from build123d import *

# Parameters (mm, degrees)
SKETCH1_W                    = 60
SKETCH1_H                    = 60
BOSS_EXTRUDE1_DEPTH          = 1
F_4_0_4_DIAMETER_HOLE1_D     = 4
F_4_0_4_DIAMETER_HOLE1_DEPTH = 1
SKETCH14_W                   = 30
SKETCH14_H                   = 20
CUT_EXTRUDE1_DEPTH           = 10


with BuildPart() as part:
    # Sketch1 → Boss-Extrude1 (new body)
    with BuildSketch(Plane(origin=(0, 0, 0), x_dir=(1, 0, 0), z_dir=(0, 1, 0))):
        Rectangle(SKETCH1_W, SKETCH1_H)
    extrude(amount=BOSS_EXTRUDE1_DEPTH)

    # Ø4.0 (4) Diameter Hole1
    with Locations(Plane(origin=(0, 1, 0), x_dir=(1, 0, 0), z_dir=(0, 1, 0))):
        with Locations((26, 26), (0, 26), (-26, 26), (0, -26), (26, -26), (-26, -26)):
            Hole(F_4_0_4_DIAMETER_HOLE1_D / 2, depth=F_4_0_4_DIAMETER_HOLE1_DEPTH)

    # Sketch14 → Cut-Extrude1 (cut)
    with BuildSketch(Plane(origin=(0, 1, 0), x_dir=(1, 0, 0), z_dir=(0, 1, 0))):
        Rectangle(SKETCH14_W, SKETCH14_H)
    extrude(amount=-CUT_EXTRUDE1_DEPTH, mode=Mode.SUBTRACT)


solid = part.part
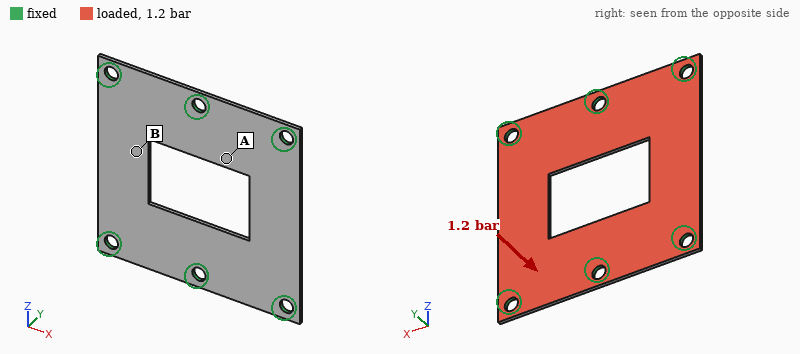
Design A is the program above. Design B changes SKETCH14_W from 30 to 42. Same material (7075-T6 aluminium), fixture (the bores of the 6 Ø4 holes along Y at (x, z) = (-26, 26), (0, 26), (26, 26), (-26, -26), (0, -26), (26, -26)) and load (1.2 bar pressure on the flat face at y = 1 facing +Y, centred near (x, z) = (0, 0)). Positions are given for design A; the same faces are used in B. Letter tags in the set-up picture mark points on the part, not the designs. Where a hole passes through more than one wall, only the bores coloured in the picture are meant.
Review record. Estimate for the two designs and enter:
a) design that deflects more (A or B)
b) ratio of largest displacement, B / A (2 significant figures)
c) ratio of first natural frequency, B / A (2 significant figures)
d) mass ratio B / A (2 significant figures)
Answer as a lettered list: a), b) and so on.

a) A
b) 0.88
c) 1.1
d) 0.92
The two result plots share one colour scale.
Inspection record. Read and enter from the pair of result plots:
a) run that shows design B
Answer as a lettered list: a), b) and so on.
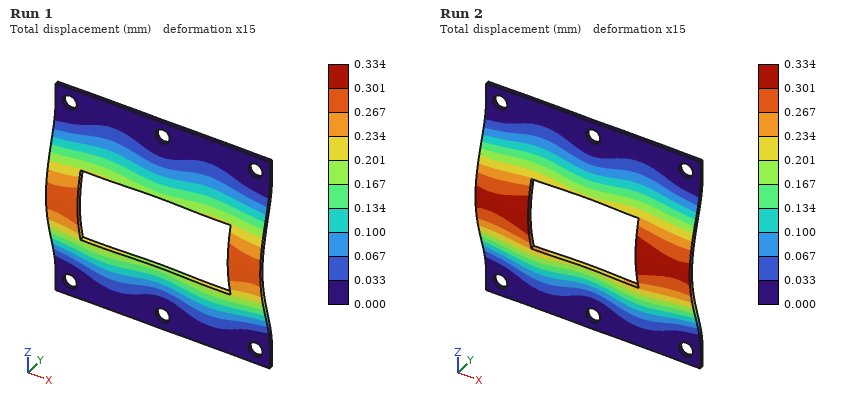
a) Run 1
